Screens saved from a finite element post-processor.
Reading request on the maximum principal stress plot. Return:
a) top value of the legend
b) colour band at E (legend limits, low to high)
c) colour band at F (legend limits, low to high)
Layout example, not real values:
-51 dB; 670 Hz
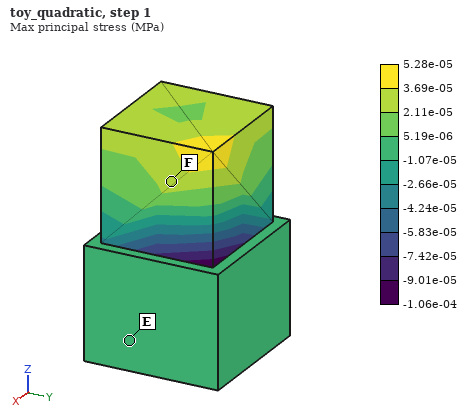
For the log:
5.28e-05 MPa; -1.07e-05 to 5.19e-06 MPa; 2.11e-05 to 3.69e-05 MPa
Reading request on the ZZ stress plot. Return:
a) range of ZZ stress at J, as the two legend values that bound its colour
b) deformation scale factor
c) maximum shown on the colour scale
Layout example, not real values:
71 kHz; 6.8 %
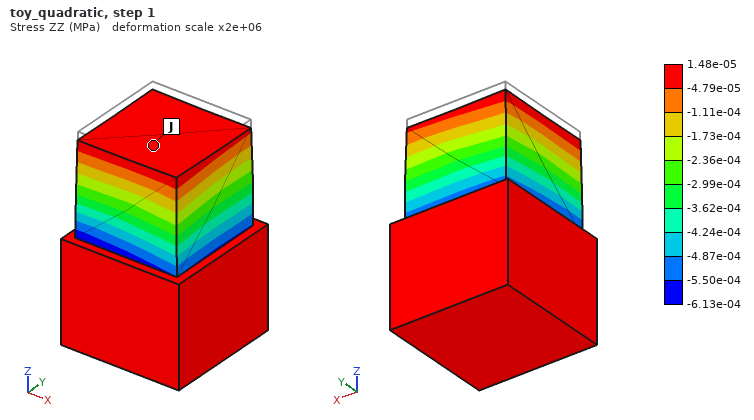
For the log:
-4.79e-05 to 1.48e-05 MPa; 2e+06; 1.48e-05 MPa
